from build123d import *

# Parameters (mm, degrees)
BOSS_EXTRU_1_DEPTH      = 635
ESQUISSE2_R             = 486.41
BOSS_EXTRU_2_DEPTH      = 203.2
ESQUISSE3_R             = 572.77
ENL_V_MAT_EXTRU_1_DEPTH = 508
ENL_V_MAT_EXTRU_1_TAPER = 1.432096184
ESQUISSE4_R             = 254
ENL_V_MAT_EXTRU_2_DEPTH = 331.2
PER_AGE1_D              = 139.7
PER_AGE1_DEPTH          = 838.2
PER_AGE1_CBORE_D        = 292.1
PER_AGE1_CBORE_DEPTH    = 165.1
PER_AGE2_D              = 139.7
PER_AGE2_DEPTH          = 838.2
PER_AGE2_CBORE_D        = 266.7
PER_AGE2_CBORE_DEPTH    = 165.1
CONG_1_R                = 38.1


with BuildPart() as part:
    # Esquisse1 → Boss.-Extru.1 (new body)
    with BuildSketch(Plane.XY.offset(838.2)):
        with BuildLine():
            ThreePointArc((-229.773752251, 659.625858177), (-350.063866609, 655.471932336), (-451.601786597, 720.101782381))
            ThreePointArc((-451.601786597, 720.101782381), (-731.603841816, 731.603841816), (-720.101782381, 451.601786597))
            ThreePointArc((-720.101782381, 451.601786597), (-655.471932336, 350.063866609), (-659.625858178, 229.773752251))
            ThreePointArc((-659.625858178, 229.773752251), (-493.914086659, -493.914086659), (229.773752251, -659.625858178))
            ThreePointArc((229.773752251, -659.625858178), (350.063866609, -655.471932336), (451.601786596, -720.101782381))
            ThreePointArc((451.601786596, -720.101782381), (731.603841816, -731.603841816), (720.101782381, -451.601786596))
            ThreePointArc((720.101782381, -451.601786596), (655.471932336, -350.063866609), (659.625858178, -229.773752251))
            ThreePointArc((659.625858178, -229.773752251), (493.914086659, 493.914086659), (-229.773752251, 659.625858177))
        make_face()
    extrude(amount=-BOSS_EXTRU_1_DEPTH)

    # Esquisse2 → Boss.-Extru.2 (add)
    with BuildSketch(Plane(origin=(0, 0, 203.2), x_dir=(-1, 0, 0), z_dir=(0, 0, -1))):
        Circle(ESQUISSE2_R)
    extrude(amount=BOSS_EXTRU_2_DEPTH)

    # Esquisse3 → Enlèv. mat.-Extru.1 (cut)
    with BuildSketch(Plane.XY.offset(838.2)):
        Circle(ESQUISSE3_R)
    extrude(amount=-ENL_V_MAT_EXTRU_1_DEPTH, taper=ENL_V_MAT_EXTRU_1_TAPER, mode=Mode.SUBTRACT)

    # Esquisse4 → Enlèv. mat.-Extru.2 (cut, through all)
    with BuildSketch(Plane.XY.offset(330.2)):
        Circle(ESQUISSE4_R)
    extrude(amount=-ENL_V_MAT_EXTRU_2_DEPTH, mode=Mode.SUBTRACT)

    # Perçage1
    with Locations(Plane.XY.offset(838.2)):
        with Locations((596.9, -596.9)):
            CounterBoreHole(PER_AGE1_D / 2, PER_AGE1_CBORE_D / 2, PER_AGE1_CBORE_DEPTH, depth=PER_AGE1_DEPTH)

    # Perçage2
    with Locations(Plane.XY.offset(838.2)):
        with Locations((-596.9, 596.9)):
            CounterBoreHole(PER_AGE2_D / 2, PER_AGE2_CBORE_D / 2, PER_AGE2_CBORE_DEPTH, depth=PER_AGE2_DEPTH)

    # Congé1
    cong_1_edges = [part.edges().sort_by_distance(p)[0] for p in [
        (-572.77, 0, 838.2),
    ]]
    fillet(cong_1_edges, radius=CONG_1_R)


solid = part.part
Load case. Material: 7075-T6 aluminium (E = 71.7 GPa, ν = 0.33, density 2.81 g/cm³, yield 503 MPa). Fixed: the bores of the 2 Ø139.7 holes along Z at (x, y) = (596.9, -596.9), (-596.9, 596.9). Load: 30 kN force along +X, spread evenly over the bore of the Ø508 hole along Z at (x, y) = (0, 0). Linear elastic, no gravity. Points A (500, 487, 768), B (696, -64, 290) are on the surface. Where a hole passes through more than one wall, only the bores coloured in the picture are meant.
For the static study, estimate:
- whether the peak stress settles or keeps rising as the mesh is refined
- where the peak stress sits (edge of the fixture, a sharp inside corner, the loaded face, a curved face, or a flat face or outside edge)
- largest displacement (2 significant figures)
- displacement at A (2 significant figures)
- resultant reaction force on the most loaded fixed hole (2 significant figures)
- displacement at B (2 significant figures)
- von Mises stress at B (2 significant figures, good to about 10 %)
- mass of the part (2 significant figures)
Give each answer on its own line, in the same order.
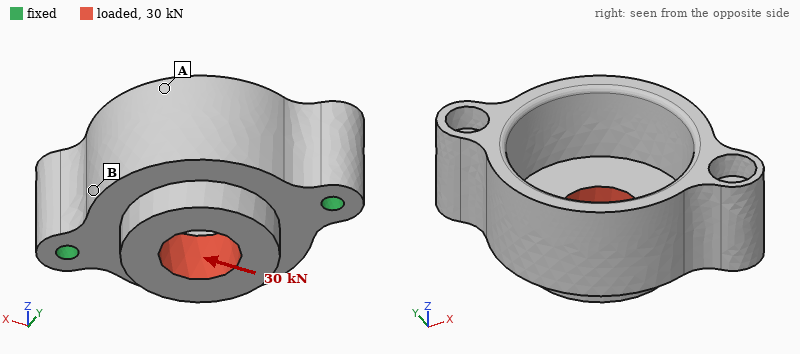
keeps rising
edge of the fixture
4.8 µm
3.9 µm
15 kN
3.1 µm
0.12 MPa
1900 kg
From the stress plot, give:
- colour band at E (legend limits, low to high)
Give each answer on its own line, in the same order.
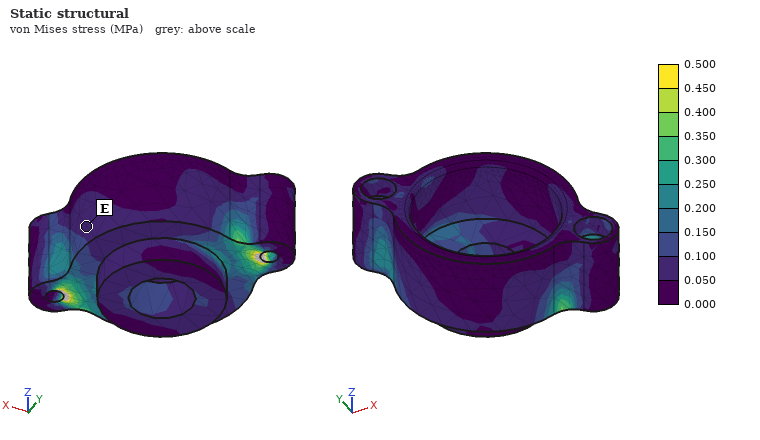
0.050 to 0.100 MPa
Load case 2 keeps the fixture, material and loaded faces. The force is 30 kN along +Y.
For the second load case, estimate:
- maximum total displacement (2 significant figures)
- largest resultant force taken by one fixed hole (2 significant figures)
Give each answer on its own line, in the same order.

4.8 µm
15 kN
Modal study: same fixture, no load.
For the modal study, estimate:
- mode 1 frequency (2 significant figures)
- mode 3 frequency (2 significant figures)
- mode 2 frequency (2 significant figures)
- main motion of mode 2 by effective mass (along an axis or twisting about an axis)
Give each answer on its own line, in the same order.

300 Hz
510 Hz
410 Hz
along Z
